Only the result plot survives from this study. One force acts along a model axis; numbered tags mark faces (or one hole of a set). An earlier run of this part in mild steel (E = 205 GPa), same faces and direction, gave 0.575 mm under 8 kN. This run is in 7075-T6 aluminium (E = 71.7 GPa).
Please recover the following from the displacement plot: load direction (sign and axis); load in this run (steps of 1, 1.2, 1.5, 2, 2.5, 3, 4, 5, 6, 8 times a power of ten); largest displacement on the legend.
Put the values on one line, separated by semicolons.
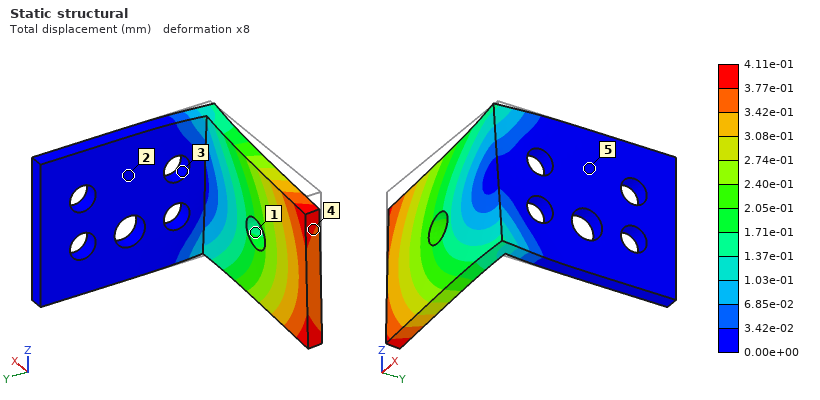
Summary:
-Z; 2 kN; 4.11e-01 mm
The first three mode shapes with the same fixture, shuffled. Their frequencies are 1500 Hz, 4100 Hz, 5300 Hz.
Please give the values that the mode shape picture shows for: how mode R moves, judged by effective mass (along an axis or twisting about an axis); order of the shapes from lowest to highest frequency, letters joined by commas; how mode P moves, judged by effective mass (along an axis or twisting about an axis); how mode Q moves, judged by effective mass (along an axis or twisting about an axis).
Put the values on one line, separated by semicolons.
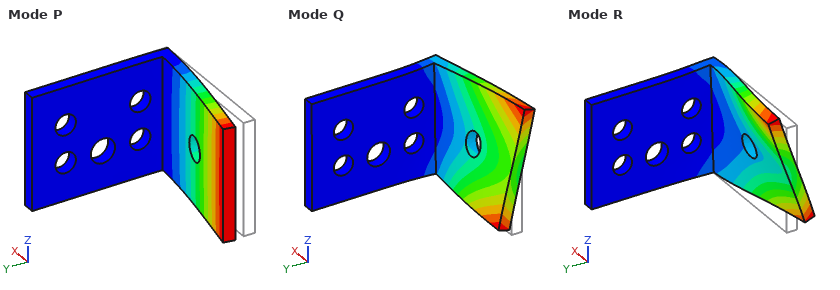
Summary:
along Z; P, Q, R; along Y; along Z
